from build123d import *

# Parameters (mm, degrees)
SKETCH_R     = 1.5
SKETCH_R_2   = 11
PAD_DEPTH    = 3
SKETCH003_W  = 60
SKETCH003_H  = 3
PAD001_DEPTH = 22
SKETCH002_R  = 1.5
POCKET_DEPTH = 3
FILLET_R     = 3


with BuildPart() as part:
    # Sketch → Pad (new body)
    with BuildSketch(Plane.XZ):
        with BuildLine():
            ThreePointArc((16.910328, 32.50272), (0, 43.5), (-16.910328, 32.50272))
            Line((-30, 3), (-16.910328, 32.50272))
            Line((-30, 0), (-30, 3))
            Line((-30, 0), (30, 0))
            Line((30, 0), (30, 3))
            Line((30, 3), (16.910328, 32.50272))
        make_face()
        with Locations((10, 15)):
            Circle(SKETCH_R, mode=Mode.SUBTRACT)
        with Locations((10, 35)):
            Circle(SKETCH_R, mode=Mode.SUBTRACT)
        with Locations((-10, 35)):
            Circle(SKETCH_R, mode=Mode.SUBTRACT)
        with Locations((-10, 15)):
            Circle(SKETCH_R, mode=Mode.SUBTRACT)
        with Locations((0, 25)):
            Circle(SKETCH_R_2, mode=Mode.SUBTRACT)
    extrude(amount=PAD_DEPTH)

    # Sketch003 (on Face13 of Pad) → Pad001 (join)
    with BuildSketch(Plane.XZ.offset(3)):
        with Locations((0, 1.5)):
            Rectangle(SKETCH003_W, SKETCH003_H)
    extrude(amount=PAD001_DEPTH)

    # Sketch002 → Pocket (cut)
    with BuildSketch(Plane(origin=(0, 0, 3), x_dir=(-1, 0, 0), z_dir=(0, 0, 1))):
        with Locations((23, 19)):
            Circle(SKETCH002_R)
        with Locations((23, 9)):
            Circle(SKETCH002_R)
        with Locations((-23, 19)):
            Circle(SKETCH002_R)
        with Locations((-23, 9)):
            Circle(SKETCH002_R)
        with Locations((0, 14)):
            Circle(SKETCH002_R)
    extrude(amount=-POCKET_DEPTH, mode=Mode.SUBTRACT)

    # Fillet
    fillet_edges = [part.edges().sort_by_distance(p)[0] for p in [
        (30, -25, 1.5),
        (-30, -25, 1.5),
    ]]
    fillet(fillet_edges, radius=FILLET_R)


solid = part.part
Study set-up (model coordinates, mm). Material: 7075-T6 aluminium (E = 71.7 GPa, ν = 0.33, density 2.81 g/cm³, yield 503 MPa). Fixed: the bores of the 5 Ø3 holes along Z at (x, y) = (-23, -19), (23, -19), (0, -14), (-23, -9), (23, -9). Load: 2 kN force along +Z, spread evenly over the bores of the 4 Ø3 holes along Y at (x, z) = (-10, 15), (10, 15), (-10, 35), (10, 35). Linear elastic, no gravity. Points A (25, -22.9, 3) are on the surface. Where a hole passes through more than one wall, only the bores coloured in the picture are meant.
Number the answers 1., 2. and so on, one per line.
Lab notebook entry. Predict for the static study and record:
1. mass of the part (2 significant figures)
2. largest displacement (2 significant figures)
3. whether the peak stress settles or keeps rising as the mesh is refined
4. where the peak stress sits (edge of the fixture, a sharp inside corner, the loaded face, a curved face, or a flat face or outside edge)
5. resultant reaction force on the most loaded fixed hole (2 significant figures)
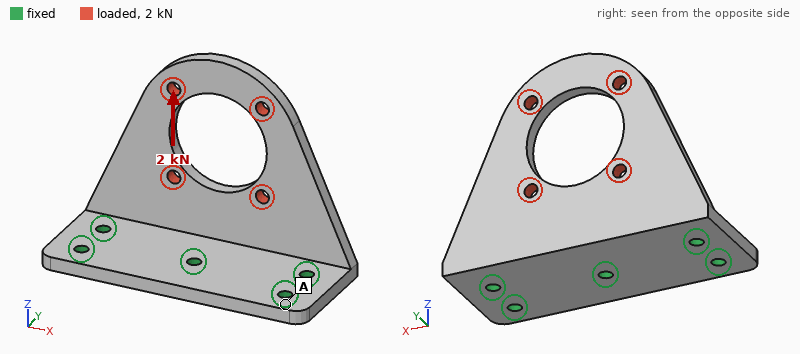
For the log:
1. 23 g
2. 0.33 mm
3. keeps rising
4. edge of the fixture
5. 1.1 kN
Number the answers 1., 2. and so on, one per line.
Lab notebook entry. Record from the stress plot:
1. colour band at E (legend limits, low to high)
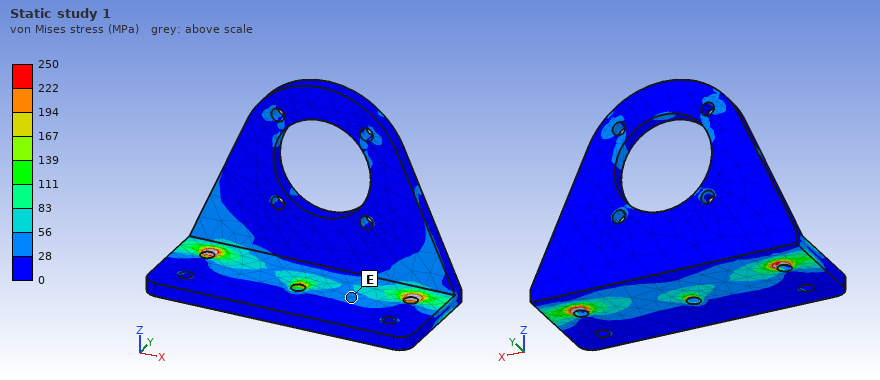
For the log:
1. 28 to 56 MPa
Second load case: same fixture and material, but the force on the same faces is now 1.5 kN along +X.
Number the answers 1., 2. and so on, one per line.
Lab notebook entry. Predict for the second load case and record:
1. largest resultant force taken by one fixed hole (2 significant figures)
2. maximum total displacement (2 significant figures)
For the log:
1. 1.0 kN
2. 0.12 mm
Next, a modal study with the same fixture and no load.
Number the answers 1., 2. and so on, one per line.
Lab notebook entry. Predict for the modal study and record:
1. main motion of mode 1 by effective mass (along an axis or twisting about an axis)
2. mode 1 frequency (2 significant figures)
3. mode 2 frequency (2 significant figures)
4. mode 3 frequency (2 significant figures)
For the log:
1. along Y
2. 1600 Hz
3. 4100 Hz
4. 6400 Hz
